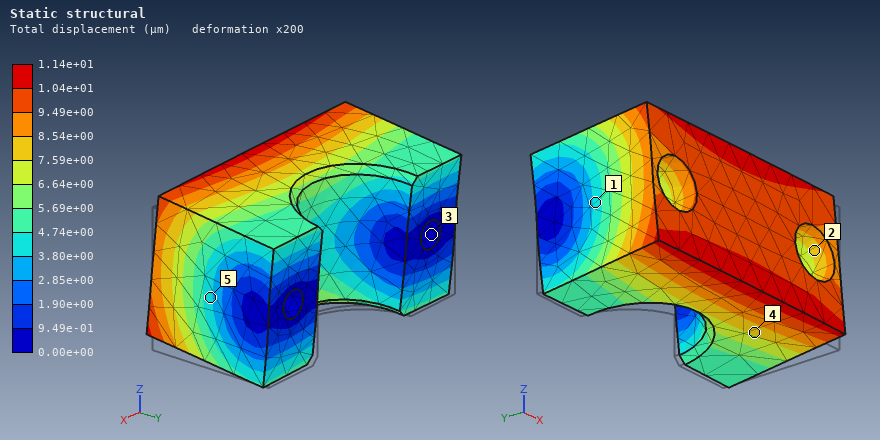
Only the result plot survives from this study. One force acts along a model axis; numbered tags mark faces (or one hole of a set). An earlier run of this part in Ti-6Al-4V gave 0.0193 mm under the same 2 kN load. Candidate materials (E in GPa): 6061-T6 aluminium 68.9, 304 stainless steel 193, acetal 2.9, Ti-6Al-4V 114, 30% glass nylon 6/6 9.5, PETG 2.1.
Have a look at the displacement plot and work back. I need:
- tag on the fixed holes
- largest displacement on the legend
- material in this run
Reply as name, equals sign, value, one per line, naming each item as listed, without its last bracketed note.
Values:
tag on the fixed holes = 3
largest displacement on the legend = 1.14e+01 µm
material in this run = 304 stainless steel
